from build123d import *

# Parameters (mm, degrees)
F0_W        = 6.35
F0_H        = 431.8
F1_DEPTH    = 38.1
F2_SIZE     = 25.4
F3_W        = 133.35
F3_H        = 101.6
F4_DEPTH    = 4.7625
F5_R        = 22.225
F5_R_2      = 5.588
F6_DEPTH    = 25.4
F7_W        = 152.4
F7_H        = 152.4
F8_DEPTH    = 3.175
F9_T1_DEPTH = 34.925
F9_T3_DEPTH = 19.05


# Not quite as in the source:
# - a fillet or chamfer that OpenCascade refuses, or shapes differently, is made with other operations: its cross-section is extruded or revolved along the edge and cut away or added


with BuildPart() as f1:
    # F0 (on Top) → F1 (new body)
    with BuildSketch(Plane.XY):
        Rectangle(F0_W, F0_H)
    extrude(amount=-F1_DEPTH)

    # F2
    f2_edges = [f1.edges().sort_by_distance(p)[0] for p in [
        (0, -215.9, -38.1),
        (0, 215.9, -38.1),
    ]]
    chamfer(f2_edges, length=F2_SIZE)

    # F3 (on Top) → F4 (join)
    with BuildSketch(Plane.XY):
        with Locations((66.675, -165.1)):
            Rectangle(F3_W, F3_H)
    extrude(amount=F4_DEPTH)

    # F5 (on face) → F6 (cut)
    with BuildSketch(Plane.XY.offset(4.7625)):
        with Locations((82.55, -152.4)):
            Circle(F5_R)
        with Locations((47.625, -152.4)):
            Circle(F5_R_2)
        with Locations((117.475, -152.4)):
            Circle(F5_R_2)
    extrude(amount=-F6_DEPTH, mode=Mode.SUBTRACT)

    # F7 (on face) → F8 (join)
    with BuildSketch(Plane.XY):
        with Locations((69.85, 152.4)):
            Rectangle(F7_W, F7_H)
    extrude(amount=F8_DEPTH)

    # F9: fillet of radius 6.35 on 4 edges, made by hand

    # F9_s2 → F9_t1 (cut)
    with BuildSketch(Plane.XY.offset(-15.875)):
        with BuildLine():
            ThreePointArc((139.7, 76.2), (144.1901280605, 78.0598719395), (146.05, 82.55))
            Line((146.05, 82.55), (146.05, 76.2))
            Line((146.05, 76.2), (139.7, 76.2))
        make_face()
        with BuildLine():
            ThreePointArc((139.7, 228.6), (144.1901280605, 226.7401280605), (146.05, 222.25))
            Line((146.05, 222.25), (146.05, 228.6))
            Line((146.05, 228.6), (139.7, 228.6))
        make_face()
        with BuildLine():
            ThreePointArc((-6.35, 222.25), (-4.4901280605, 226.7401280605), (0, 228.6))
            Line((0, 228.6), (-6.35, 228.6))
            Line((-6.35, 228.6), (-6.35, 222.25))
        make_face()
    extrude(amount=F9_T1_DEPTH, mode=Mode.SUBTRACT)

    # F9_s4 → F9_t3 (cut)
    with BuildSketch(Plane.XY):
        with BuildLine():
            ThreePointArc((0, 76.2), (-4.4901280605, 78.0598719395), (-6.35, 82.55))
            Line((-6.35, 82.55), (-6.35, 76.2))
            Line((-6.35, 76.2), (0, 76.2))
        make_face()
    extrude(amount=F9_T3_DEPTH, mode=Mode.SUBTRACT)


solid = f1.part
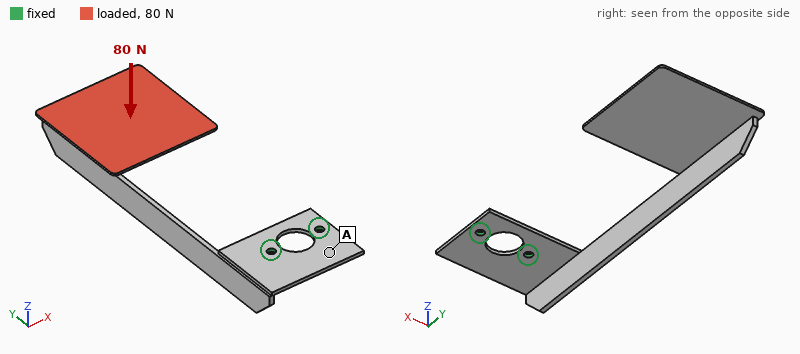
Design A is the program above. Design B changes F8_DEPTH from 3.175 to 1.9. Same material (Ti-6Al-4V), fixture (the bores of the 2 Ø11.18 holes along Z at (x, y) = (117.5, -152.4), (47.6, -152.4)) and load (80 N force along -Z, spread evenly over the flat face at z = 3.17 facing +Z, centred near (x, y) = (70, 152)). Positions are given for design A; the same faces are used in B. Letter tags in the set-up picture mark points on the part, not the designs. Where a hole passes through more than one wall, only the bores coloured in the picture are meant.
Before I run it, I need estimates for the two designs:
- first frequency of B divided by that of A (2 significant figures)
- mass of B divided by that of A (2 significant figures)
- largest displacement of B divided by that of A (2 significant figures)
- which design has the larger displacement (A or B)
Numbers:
1.2
0.87
1.4
B
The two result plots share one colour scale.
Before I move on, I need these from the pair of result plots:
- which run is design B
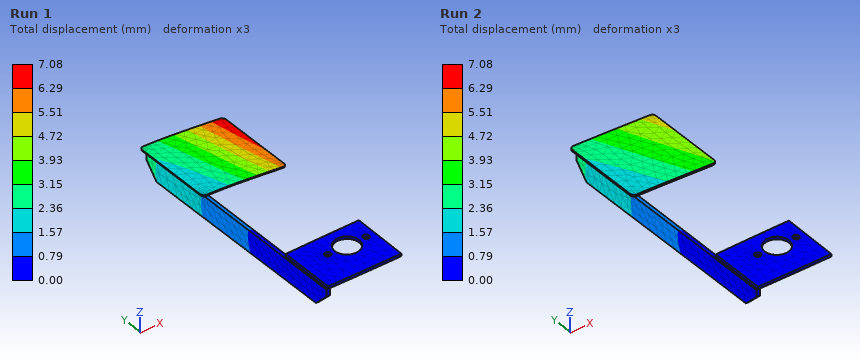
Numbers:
Run 1
